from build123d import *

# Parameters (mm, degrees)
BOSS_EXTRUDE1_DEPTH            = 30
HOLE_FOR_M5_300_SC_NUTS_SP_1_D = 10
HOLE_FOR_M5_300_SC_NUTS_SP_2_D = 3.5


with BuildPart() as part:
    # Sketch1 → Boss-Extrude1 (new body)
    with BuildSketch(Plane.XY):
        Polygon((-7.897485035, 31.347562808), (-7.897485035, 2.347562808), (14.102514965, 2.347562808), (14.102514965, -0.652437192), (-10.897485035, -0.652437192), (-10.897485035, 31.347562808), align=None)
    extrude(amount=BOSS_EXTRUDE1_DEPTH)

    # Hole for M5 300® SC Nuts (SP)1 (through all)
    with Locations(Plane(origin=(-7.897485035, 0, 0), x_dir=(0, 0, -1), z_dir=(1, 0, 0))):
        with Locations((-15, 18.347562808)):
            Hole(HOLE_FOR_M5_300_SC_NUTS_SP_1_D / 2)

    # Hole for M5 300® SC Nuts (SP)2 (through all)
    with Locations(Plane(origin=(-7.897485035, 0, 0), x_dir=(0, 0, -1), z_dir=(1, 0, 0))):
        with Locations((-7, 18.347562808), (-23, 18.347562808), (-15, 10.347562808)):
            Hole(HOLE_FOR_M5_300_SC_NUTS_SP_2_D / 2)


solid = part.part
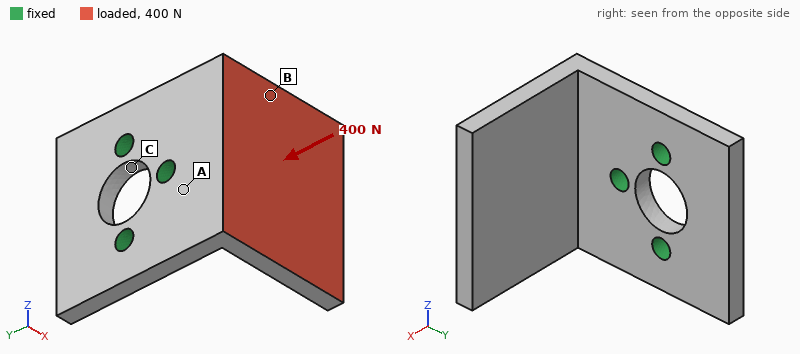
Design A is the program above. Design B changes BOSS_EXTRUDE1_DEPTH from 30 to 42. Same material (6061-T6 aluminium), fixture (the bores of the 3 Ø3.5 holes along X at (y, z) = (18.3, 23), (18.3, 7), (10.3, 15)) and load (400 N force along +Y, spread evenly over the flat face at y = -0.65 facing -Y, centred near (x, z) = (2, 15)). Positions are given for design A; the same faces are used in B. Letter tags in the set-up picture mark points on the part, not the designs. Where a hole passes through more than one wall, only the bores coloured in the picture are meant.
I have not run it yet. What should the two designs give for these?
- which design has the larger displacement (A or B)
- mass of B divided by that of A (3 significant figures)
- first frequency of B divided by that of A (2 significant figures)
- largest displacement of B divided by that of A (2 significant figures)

A
1.43
0.90
0.82
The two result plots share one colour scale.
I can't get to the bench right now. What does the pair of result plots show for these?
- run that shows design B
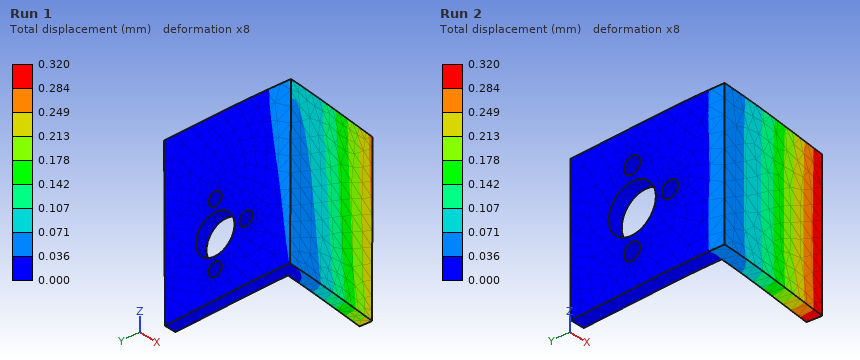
Run 1
